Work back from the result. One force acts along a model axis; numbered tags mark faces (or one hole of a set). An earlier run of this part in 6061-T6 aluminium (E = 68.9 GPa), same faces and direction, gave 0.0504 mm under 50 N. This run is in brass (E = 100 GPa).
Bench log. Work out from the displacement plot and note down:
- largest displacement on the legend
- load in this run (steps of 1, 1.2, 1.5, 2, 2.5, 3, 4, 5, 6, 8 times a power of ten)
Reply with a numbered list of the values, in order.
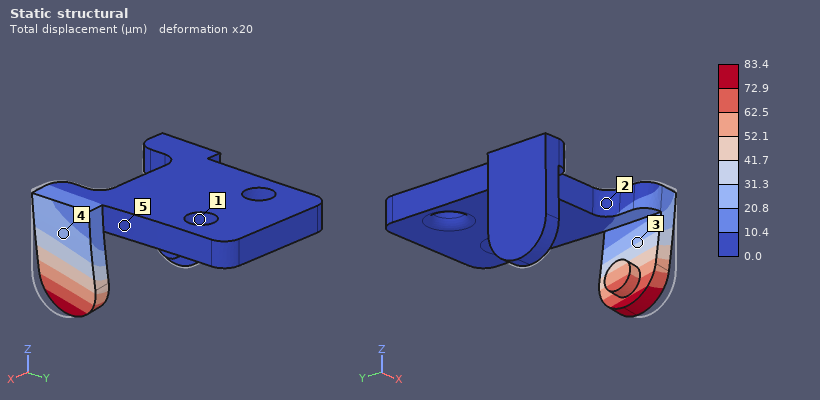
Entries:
1. 83.4 µm
2. 120 N
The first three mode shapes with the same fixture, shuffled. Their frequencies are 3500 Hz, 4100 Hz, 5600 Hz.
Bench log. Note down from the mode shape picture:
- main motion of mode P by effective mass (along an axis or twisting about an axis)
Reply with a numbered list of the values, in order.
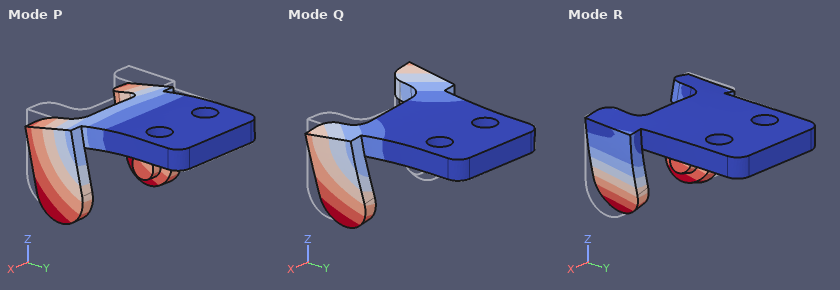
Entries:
1. along Z
